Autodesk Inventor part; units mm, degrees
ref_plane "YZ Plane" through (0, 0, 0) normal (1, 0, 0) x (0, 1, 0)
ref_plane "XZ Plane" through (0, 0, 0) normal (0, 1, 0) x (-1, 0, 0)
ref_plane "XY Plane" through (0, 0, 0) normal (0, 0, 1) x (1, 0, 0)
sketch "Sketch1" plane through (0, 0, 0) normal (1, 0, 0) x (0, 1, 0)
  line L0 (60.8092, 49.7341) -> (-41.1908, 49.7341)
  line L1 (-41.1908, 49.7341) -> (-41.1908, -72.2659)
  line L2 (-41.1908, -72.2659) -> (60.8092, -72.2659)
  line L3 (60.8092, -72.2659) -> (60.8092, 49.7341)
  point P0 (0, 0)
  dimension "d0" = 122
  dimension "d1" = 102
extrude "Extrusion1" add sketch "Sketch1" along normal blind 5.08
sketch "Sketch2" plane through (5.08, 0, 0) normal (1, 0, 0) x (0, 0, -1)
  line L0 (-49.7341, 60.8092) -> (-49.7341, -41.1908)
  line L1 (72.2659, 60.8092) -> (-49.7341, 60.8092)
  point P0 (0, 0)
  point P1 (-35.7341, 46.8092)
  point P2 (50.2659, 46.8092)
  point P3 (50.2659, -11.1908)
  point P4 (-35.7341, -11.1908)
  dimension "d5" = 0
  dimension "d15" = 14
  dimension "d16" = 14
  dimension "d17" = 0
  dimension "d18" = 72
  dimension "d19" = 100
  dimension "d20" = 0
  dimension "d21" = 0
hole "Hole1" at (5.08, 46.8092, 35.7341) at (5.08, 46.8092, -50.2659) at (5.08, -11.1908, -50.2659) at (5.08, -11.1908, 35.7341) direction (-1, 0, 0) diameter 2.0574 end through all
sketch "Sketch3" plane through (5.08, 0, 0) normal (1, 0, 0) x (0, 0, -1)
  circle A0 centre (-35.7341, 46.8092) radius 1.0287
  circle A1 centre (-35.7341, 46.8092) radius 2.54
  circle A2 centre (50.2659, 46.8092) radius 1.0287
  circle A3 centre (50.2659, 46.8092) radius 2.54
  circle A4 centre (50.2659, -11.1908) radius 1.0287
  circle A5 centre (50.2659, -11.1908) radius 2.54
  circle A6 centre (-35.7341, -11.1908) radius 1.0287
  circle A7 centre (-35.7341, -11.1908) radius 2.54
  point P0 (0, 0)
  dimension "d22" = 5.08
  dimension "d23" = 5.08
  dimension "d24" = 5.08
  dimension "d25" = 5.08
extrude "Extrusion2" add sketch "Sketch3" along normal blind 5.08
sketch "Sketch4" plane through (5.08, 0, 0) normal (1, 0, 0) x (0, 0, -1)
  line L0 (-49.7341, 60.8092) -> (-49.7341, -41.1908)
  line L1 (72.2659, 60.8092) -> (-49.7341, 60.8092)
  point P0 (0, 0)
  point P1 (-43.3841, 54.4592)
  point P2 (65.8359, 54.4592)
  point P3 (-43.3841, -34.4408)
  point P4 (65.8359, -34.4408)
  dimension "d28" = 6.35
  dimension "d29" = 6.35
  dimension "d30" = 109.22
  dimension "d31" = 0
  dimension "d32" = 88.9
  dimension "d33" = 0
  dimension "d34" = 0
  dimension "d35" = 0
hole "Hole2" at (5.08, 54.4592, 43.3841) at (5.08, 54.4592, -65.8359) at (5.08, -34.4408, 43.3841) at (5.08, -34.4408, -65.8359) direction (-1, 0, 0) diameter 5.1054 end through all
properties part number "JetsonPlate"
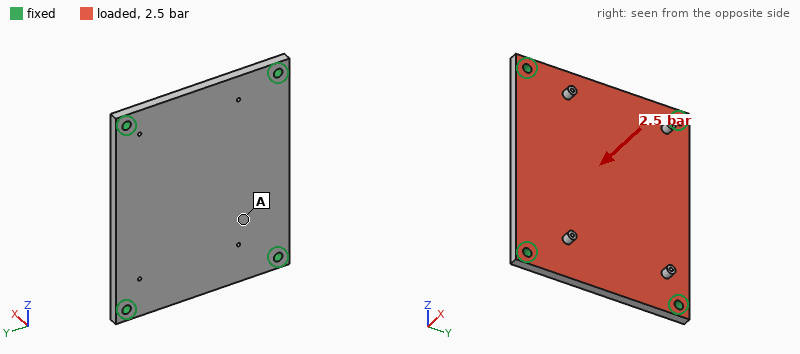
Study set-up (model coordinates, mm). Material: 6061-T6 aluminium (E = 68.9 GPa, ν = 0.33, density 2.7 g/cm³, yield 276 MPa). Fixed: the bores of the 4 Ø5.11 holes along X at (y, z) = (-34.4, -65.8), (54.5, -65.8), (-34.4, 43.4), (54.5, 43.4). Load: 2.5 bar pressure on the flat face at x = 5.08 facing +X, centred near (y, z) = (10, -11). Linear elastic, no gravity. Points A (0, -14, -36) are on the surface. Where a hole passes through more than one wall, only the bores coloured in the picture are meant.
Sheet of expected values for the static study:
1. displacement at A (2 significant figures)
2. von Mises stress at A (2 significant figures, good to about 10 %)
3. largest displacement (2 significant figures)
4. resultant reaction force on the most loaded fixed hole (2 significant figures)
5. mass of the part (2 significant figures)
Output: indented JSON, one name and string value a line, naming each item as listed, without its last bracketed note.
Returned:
{
  "displacement at A": "0.17 mm",
  "von Mises stress at A": "22 MPa",
  "largest displacement": "0.25 mm",
  "resultant reaction force on the most loaded fixed hole": "770 N",
  "mass of the part": "170 g"
}
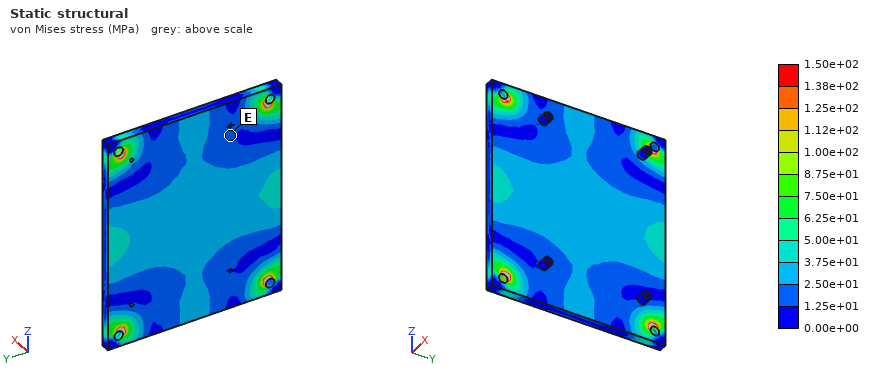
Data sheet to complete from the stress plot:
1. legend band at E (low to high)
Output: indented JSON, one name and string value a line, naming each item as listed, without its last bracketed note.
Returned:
{
  "legend band at E": "1.25e+01 to 2.50e+01 MPa"
}
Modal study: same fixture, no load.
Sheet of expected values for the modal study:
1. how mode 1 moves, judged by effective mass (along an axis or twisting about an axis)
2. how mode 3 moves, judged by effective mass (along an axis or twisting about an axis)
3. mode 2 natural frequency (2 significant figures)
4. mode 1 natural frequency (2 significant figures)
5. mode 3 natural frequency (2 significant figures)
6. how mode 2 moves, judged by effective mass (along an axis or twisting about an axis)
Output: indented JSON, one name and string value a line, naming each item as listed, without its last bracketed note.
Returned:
{
  "how mode 1 moves, judged by effective mass": "along X",
  "how mode 3 moves, judged by effective mass": "twisting about Y",
  "mode 2 natural frequency": "2600 Hz",
  "mode 1 natural frequency": "1600 Hz",
  "mode 3 natural frequency": "3300 Hz",
  "how mode 2 moves, judged by effective mass": "twisting about Z"
}
